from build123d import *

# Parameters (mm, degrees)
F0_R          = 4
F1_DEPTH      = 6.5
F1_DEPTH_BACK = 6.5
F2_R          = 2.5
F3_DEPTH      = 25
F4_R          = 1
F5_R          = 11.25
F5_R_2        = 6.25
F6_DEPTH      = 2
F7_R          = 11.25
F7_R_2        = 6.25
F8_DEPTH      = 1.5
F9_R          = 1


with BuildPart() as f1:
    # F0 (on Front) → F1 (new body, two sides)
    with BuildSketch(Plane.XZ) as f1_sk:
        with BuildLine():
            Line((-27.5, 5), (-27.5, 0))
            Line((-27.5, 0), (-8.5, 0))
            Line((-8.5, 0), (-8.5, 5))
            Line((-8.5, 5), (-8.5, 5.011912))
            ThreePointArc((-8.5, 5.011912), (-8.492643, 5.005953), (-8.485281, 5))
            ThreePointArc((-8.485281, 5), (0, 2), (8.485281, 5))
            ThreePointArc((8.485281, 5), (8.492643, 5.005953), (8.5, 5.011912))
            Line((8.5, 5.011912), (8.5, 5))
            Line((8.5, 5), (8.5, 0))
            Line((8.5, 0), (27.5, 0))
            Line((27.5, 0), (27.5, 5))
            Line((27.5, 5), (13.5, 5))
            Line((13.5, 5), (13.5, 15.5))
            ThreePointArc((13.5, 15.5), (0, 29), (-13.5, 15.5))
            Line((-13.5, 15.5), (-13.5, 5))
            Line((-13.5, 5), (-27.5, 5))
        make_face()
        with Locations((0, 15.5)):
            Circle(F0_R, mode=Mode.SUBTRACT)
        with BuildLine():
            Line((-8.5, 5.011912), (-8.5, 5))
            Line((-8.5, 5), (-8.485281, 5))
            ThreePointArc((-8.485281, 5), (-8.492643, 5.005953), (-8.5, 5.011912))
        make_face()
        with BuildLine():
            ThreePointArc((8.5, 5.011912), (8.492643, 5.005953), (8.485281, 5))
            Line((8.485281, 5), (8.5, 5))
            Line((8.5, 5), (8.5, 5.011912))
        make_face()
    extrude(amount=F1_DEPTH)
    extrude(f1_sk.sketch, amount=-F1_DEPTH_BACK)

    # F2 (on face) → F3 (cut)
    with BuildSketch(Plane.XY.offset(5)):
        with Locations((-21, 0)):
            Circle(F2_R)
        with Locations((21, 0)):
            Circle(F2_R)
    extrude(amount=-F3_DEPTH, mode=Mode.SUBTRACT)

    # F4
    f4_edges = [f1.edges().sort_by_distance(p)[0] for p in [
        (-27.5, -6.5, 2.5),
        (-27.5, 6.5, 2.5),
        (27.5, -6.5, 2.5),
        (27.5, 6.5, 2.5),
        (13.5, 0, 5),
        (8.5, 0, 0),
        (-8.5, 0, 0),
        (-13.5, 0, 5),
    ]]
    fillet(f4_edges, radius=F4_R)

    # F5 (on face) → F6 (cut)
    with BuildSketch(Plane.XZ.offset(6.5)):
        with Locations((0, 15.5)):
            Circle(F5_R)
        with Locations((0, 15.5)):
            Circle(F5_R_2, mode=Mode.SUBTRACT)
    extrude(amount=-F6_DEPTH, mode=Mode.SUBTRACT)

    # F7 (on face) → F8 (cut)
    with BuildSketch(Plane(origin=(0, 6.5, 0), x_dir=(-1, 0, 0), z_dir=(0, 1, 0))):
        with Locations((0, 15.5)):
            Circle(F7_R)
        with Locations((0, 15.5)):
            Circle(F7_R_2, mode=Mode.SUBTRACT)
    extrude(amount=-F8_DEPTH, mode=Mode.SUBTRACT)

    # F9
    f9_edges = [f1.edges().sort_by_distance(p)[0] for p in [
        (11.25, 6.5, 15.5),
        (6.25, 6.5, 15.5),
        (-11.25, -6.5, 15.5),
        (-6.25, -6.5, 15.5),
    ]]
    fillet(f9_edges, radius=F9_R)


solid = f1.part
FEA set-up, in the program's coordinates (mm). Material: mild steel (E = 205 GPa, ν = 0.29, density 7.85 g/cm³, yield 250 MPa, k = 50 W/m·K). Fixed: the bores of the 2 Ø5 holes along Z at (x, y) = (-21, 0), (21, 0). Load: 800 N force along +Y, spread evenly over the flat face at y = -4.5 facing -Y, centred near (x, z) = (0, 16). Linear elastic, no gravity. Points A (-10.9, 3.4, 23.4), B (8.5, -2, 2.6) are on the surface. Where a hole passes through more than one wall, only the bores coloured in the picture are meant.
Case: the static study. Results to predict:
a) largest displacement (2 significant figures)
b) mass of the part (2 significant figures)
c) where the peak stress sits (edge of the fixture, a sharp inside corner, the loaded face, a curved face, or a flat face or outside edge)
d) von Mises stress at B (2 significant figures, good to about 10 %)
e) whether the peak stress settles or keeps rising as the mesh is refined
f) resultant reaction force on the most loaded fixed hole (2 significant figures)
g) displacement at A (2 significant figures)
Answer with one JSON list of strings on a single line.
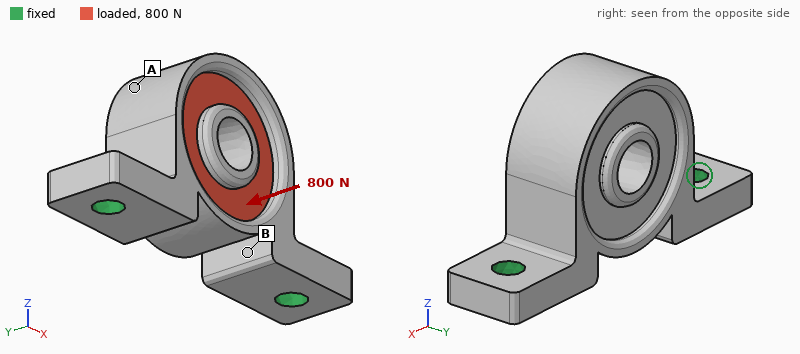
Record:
["32 µm", "66 g", "edge of the fixture", "24 MPa", "keeps rising", "400 N", "25 µm"]
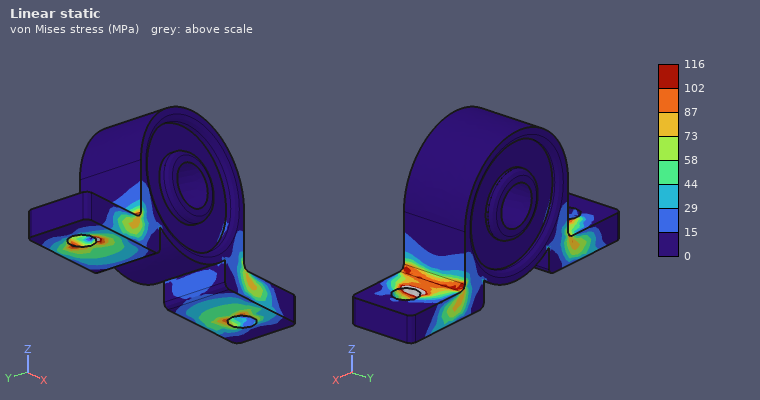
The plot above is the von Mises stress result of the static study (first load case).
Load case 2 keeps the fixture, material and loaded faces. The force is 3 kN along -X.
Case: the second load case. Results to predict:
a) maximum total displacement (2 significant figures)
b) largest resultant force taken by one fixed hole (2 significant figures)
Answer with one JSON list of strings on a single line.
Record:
["14 µm", "1.9 kN"]
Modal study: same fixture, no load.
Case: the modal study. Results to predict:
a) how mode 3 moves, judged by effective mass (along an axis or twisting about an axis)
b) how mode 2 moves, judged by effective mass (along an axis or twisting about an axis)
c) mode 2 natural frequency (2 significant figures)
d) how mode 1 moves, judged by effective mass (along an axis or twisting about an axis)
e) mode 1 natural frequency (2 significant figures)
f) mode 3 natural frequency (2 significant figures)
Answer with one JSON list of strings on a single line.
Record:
["along Z", "along X", "14 kHz", "along Y", "4600 Hz", "14 kHz"]
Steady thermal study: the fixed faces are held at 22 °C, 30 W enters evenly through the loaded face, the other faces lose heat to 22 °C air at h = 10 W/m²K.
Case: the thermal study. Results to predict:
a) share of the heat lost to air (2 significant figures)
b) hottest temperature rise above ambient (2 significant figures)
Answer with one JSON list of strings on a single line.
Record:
["5.9 %", "79 K"]
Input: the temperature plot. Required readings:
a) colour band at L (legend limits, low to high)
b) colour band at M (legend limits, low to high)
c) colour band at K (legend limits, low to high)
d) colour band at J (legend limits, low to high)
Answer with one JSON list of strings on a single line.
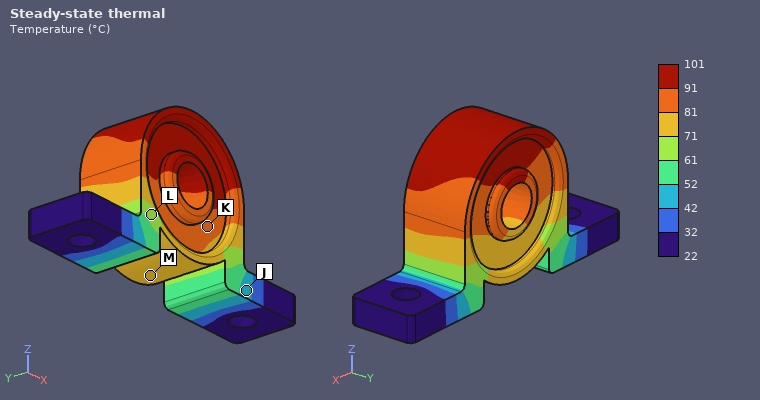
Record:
["61 to 71 °C", "71 to 81 °C", "81 to 91 °C", "42 to 52 °C"]
